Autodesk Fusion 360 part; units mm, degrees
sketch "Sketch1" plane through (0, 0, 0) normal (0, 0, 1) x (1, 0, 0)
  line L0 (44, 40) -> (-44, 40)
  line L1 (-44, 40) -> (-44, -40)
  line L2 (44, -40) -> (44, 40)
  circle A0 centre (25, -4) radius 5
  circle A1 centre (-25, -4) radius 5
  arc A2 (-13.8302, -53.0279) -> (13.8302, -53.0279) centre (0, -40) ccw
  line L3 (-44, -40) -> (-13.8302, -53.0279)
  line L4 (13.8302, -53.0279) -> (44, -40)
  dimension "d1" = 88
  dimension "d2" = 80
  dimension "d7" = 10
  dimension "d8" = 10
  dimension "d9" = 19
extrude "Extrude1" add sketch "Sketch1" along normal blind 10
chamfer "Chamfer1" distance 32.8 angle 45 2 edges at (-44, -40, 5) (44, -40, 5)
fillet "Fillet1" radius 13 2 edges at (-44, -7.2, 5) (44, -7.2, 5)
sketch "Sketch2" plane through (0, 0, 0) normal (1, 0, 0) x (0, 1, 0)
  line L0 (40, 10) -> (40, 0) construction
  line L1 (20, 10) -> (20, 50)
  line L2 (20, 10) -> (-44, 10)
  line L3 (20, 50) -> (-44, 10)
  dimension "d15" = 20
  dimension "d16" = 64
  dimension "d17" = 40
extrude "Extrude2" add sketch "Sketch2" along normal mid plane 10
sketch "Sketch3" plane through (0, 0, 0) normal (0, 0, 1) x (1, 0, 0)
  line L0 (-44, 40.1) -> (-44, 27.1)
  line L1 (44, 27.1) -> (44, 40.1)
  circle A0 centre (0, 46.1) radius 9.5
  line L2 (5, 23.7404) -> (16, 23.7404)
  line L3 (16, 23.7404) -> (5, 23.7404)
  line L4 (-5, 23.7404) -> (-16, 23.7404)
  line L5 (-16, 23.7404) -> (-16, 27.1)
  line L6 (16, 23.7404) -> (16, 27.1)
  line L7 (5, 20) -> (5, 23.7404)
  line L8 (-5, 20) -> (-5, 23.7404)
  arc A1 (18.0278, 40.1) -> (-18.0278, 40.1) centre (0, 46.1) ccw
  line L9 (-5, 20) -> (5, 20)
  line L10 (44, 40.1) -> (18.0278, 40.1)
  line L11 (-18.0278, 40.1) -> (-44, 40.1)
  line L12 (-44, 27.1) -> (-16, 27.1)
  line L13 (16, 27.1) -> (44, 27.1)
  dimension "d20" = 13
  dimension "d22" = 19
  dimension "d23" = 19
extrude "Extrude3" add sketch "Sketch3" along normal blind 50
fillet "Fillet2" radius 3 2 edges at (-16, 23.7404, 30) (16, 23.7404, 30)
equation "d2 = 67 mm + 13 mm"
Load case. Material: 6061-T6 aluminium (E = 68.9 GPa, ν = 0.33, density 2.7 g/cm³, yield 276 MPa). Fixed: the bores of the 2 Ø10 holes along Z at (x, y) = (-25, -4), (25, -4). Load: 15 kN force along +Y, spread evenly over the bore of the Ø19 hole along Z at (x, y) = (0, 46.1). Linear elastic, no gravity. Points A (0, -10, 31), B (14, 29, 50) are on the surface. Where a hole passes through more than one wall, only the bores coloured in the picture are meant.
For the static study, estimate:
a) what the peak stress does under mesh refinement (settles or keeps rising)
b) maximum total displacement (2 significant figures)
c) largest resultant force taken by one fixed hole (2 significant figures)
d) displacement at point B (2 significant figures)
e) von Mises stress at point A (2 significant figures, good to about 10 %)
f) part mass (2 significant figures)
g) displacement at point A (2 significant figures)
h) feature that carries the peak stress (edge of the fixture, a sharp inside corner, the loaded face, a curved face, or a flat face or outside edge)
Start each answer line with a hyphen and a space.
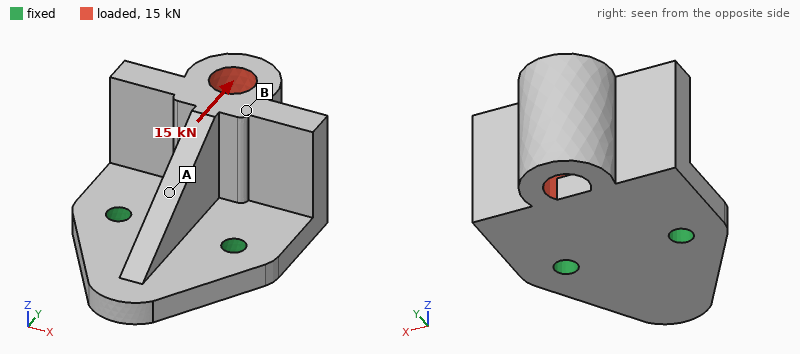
- keeps rising
- 0.45 mm
- 7.5 kN
- 0.30 mm
- 58 MPa
- 430 g
- 0.14 mm
- edge of the fixture
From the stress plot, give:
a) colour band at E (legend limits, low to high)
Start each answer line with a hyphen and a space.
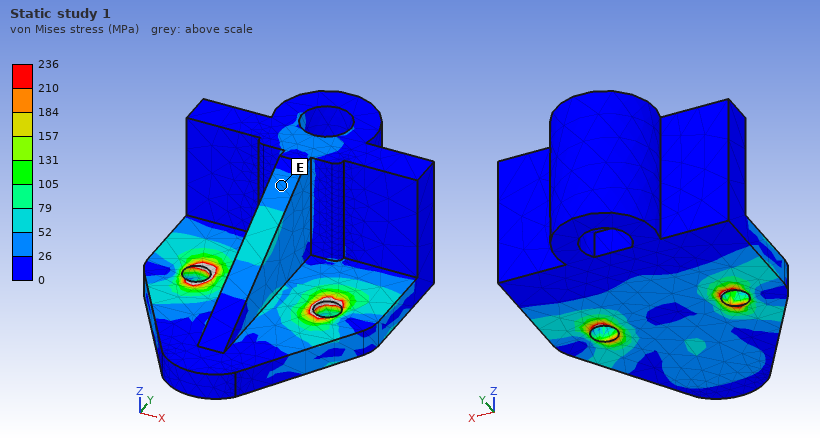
- 26 to 52 MPa
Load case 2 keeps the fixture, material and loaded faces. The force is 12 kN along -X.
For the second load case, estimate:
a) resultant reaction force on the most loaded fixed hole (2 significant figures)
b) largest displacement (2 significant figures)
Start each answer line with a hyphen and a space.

- 13 kN
- 0.18 mm
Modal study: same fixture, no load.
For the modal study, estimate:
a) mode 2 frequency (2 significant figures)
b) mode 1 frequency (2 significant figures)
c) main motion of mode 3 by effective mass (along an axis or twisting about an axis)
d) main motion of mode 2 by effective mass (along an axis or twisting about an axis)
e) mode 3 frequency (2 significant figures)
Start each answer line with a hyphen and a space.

- 2800 Hz
- 1600 Hz
- along Z
- along X
- 5400 Hz
